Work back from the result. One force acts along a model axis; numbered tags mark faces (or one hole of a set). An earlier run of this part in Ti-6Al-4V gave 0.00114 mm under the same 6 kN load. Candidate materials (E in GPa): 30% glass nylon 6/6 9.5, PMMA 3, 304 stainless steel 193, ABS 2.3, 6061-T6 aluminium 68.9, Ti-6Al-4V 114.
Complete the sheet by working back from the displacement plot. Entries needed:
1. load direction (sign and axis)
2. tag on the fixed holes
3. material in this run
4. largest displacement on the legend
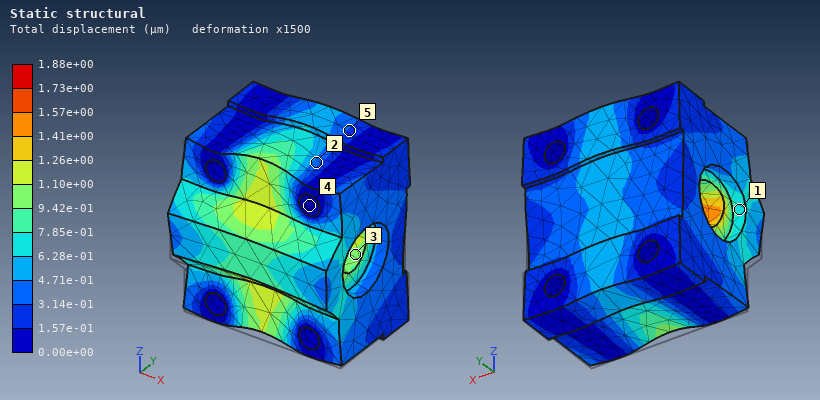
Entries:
+Z
4
6061-T6 aluminium
1.88e+00 µm
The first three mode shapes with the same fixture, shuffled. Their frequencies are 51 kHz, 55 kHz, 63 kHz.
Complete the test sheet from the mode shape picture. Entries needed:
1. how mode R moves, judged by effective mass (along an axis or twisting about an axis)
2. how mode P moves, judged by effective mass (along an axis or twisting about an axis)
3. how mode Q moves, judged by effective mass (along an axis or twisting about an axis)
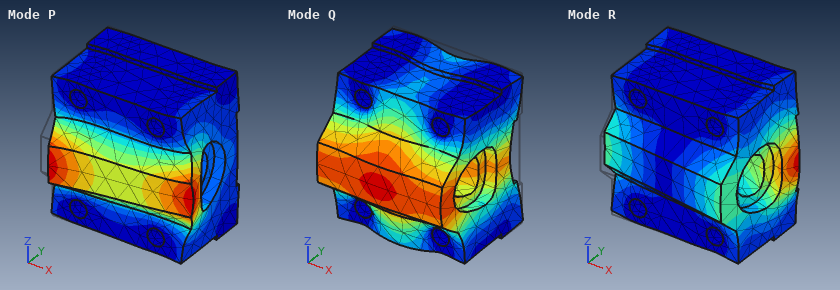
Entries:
along X
along X
along Y
